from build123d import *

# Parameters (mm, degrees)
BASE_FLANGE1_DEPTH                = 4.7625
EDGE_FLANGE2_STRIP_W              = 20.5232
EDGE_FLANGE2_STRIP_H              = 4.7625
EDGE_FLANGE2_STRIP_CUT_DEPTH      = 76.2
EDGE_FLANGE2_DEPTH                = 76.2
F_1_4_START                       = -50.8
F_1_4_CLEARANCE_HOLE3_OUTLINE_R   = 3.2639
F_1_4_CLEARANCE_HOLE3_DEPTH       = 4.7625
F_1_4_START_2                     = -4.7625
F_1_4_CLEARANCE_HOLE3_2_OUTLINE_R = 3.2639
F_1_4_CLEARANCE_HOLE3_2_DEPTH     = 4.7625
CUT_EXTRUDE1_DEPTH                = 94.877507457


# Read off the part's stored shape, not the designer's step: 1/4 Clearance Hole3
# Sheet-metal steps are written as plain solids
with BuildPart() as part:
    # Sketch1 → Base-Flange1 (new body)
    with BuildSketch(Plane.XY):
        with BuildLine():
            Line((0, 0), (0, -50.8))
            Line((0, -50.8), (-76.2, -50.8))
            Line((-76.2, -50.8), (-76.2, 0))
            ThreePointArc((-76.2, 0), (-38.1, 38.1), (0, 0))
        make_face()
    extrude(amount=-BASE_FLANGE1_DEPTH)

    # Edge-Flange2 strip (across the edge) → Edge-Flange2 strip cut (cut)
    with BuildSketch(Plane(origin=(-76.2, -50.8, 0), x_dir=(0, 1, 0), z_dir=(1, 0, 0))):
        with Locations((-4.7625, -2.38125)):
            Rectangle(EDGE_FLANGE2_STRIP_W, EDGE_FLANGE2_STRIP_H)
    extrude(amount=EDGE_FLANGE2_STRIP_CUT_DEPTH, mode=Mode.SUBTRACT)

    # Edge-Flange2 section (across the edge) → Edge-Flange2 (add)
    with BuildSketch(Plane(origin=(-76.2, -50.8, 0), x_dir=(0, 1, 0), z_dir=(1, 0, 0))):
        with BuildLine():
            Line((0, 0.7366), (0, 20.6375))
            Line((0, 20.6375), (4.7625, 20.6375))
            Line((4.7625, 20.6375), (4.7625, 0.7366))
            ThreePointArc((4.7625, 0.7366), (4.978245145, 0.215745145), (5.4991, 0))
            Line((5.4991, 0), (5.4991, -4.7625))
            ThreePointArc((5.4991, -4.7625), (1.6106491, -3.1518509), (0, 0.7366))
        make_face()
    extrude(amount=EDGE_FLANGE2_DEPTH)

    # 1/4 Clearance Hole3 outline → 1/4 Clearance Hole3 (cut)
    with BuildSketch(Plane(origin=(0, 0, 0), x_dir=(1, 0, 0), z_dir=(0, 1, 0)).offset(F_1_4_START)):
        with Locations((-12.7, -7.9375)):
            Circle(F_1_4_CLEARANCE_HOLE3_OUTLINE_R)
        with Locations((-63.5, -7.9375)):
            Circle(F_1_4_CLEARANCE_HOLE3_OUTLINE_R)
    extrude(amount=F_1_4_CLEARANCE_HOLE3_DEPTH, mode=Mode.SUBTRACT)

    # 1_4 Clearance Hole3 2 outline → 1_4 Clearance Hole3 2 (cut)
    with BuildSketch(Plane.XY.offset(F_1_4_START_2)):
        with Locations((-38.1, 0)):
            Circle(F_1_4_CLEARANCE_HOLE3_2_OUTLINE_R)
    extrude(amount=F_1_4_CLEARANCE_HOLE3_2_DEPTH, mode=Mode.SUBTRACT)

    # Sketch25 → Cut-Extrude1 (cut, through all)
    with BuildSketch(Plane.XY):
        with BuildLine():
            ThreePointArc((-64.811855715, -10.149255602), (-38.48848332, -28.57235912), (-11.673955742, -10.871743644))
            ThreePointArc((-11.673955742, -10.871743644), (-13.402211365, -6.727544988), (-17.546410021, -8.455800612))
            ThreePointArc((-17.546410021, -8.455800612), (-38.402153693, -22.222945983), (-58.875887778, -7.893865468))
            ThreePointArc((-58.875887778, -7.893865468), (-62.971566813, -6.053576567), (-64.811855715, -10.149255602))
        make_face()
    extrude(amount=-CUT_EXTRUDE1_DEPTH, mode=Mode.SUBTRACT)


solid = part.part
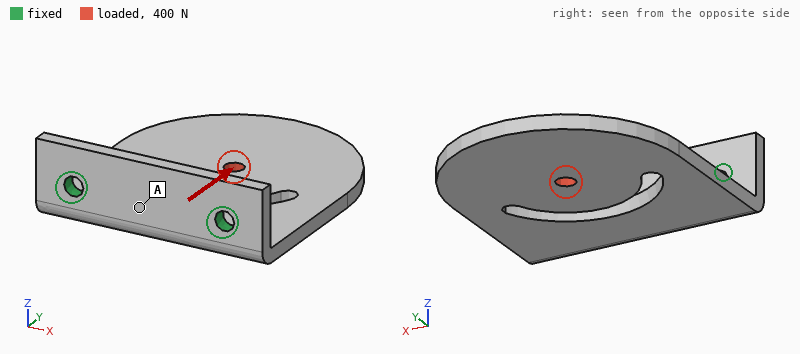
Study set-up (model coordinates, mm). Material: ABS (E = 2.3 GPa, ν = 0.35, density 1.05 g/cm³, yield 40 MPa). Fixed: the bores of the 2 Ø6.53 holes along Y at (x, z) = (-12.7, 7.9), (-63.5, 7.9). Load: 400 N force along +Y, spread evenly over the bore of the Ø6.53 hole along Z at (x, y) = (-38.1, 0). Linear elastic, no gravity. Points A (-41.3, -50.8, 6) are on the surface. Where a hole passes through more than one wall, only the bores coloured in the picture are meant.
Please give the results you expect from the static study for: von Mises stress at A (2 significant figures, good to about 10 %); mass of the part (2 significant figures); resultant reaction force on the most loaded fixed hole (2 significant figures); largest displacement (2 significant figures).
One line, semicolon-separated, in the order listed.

1.8 MPa; 36 g; 200 N; 1.2 mm
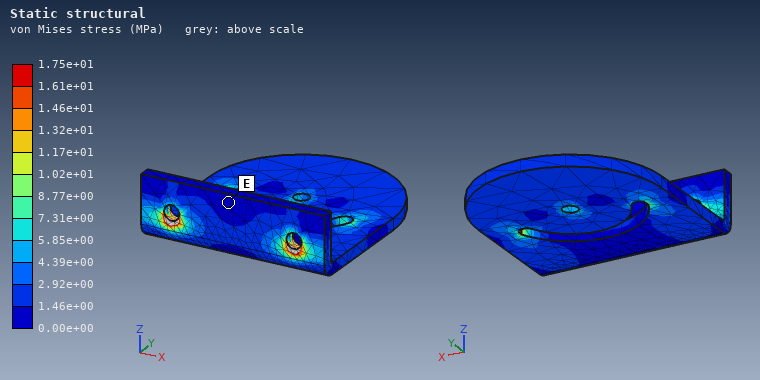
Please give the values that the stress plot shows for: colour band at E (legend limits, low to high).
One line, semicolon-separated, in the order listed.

0.00e+00 to 1.46e+00 MPa
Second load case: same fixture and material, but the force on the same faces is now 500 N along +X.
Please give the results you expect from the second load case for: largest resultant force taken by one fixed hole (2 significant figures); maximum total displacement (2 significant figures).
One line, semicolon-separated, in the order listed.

520 N; 1.4 mm
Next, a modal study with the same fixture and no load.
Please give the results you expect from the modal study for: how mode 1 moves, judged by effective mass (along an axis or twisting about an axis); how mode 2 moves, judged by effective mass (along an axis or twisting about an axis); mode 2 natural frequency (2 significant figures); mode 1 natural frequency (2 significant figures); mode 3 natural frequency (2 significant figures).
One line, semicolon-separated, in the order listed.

along Z; twisting about Y; 420 Hz; 130 Hz; 600 Hz
